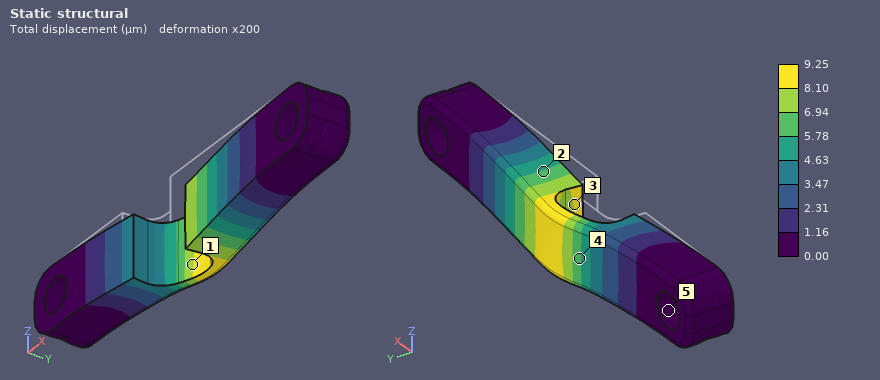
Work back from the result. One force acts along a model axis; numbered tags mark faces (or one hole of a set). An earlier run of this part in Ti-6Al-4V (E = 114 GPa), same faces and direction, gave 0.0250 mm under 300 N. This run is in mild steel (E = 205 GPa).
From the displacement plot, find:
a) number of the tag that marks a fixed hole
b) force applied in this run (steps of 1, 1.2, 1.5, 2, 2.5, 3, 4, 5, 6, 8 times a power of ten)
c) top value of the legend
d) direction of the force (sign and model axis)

5
200 N
9.25 µm
+Y
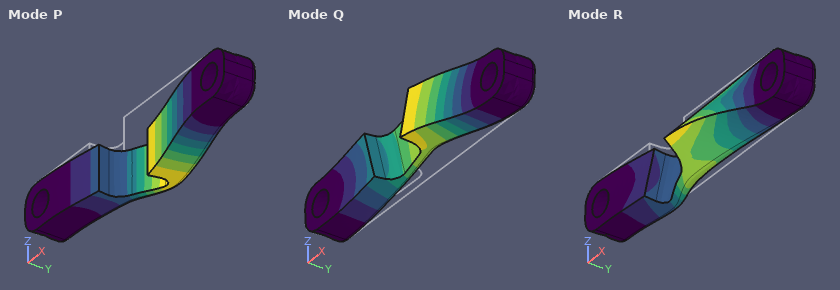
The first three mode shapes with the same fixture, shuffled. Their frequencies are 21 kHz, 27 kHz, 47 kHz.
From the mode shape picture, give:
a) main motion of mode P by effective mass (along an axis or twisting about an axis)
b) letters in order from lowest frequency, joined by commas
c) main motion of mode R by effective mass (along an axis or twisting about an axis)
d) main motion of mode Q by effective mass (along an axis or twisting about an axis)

along Y
P, Q, R
twisting about X
along Z
